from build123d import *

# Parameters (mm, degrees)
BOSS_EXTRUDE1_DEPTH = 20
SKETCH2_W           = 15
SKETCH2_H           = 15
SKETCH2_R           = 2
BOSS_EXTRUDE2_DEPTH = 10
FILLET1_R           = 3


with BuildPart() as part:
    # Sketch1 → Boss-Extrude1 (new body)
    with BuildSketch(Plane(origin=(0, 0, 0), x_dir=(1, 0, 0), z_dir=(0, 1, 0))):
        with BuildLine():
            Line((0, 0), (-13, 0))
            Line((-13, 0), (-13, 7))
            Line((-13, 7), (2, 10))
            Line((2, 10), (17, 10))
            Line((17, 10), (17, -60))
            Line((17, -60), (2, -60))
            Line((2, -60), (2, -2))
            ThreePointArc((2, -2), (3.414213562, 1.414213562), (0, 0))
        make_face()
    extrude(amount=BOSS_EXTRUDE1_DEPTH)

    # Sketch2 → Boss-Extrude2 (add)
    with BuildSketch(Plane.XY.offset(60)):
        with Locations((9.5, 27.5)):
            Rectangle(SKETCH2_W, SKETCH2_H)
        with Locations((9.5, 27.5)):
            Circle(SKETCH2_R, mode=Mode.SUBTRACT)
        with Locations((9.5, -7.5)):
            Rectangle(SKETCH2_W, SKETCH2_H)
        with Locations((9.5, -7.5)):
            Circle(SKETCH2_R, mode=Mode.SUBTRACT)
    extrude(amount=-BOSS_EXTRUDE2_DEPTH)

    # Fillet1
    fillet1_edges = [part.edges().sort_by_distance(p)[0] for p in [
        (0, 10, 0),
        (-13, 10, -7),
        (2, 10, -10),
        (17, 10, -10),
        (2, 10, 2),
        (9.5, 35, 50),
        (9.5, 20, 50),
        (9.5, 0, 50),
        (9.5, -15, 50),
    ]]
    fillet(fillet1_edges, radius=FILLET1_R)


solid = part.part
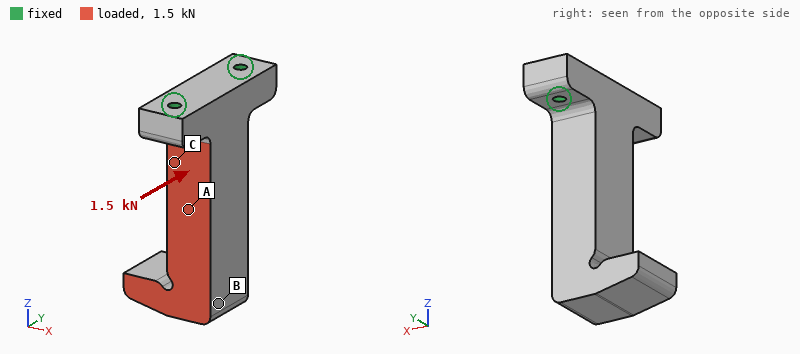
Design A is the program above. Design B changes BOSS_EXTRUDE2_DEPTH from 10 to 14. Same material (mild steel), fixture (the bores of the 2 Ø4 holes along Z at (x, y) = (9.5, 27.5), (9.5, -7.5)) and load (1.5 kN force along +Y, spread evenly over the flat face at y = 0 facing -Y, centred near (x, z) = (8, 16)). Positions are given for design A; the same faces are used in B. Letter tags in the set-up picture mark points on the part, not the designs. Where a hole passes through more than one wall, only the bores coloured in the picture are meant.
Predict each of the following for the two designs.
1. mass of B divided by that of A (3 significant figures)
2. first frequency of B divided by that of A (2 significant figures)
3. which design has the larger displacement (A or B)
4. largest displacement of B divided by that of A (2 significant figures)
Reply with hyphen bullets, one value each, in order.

- 1.06
- 1.3
- A
- 0.81
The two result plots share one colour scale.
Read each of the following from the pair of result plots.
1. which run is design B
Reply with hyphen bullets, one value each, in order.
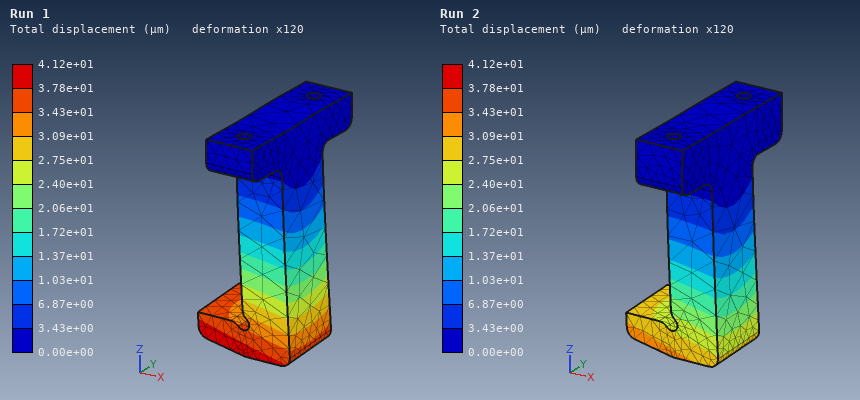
- Run 2
